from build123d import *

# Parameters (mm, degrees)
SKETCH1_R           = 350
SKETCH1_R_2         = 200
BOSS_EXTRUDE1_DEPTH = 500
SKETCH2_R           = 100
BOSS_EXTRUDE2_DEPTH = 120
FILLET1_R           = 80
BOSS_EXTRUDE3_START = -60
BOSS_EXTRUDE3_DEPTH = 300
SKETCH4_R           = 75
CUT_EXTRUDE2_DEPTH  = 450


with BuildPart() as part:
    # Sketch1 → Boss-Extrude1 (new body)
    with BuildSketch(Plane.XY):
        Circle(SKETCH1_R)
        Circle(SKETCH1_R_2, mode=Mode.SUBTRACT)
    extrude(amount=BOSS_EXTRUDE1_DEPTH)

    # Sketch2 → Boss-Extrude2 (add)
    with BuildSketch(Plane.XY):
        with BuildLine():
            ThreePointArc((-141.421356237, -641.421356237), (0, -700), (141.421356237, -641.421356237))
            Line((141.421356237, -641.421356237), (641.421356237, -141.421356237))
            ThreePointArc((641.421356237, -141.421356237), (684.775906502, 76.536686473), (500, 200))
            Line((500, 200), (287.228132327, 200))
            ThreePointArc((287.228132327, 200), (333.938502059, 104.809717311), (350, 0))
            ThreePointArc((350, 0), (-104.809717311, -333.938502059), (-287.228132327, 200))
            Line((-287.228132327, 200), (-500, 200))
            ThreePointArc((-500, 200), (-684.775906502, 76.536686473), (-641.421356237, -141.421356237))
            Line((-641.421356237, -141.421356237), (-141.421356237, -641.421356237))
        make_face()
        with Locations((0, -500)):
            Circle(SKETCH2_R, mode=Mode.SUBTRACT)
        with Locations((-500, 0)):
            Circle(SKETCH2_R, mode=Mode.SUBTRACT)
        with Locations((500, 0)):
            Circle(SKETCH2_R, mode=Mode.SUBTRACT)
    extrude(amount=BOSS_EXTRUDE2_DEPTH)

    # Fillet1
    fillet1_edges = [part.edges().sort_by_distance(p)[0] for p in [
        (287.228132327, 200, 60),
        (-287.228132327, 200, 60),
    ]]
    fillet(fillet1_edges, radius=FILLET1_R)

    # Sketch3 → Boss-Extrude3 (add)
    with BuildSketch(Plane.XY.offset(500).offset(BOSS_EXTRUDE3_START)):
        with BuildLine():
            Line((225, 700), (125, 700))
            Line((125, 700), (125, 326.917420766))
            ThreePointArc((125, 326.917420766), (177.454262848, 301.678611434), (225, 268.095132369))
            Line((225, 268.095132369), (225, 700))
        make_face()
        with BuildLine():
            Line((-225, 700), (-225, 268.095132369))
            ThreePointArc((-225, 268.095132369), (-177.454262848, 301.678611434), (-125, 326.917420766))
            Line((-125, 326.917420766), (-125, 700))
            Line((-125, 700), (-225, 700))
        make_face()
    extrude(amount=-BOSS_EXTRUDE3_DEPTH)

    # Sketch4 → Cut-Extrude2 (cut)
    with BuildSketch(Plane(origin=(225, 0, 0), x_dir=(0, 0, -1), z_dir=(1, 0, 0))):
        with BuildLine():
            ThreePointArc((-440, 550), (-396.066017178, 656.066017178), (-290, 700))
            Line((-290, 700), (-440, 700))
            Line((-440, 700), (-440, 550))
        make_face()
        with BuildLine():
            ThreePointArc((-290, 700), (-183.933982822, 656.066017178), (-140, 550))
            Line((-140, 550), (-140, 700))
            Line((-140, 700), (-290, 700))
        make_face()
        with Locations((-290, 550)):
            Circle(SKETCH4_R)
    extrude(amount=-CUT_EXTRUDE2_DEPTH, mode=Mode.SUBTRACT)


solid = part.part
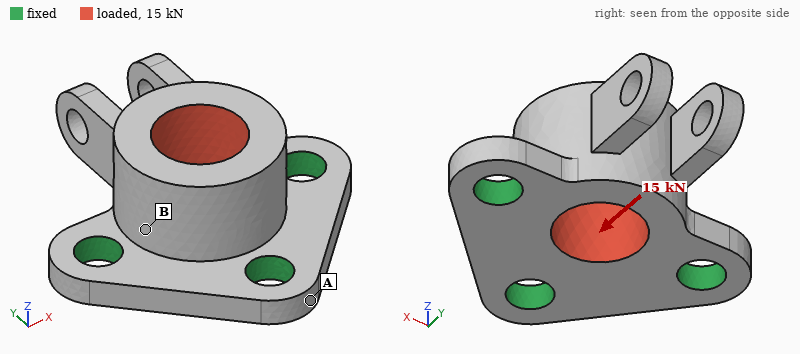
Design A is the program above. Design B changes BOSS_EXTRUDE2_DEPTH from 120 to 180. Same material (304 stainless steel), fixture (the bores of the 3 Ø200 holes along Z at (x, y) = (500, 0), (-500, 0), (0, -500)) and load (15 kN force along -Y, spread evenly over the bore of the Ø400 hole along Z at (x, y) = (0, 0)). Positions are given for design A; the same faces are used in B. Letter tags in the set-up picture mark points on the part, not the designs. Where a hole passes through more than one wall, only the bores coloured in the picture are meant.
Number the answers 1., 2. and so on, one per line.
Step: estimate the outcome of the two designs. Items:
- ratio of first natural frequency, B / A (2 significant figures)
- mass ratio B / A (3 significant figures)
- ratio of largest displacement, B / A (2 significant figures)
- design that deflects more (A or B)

1. 1.2
2. 1.13
3. 0.55
4. A
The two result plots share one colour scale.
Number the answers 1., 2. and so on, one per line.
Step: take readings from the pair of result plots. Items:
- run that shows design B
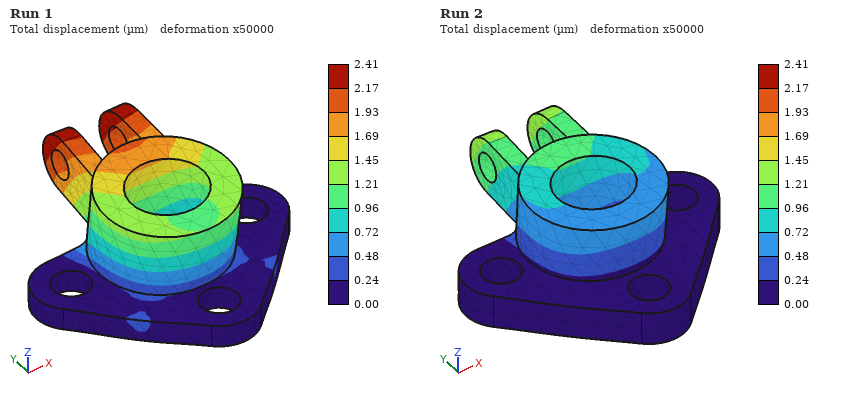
1. Run 2
